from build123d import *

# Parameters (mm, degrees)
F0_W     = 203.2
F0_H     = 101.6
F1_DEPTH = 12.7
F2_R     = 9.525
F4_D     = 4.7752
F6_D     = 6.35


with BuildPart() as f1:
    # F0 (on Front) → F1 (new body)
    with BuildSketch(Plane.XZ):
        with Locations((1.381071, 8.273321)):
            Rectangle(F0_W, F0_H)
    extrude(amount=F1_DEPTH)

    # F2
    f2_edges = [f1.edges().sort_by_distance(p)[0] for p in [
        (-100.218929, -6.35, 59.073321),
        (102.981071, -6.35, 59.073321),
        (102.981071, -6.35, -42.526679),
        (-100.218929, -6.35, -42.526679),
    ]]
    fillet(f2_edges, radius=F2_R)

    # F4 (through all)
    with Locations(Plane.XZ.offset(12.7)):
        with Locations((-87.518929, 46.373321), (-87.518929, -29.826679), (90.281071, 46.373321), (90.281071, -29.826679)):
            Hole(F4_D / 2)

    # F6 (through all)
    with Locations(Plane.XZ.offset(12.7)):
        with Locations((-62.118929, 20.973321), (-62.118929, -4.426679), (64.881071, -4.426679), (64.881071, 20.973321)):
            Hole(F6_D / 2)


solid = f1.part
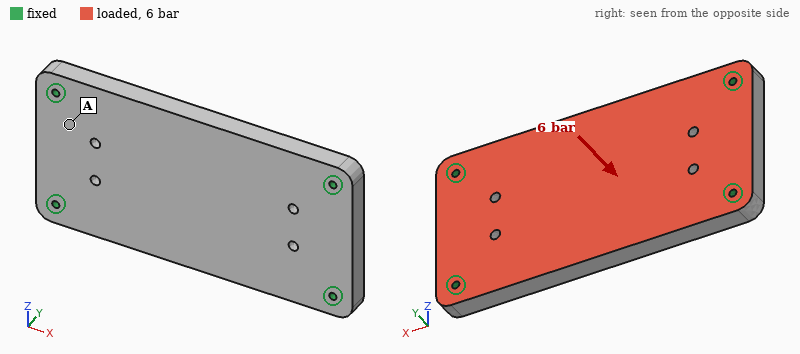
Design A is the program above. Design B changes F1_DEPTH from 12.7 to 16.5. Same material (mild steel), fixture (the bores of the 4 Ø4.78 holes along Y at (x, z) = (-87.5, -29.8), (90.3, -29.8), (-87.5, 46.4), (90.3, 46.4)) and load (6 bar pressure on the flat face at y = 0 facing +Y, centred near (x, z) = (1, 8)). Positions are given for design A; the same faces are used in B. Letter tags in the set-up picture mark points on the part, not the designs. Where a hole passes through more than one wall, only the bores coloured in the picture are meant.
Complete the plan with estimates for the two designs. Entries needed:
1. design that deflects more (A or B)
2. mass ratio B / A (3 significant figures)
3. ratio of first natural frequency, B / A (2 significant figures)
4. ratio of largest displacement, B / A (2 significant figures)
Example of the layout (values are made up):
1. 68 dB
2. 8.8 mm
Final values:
1. A
2. 1.30
3. 1.2
4. 0.50
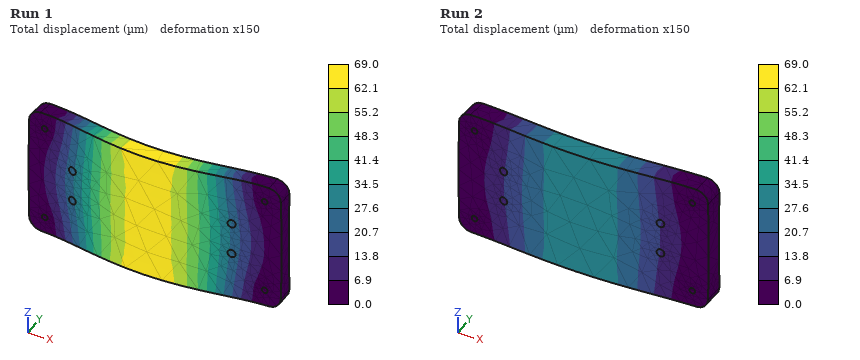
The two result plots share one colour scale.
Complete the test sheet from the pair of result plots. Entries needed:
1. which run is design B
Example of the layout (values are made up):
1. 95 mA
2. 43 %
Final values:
1. Run 2
